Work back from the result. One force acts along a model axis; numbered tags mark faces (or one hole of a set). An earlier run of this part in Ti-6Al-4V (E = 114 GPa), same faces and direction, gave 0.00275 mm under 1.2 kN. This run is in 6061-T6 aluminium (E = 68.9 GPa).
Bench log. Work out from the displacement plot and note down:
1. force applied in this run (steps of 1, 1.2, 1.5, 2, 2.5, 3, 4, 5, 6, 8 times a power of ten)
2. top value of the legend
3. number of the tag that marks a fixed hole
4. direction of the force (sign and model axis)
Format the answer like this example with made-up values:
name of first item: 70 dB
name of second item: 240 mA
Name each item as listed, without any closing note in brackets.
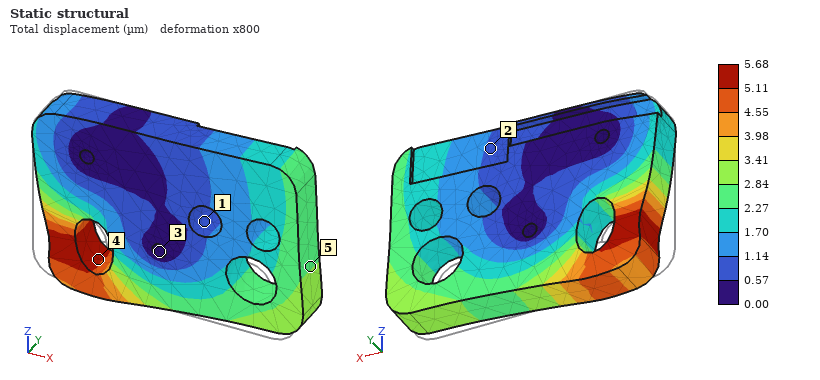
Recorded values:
force applied in this run: 1.5 kN
top value of the legend: 5.68 µm
number of the tag that marks a fixed hole: 3
direction of the force: +X
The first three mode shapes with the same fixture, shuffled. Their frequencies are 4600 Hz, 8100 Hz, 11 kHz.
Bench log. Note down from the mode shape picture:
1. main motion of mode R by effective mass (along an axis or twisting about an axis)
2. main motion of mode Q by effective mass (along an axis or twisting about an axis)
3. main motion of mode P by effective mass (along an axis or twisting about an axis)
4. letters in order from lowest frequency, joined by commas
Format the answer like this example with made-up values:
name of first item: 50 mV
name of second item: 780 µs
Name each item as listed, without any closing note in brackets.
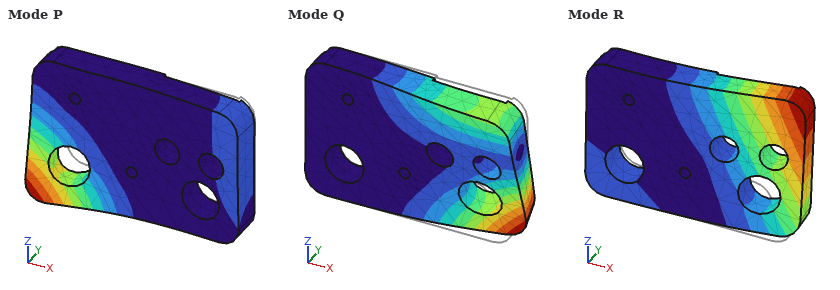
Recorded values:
main motion of mode R by effective mass: along Y
main motion of mode Q by effective mass: twisting about X
main motion of mode P by effective mass: along Y
letters in order from lowest frequency, joined by commas: R, Q, P
